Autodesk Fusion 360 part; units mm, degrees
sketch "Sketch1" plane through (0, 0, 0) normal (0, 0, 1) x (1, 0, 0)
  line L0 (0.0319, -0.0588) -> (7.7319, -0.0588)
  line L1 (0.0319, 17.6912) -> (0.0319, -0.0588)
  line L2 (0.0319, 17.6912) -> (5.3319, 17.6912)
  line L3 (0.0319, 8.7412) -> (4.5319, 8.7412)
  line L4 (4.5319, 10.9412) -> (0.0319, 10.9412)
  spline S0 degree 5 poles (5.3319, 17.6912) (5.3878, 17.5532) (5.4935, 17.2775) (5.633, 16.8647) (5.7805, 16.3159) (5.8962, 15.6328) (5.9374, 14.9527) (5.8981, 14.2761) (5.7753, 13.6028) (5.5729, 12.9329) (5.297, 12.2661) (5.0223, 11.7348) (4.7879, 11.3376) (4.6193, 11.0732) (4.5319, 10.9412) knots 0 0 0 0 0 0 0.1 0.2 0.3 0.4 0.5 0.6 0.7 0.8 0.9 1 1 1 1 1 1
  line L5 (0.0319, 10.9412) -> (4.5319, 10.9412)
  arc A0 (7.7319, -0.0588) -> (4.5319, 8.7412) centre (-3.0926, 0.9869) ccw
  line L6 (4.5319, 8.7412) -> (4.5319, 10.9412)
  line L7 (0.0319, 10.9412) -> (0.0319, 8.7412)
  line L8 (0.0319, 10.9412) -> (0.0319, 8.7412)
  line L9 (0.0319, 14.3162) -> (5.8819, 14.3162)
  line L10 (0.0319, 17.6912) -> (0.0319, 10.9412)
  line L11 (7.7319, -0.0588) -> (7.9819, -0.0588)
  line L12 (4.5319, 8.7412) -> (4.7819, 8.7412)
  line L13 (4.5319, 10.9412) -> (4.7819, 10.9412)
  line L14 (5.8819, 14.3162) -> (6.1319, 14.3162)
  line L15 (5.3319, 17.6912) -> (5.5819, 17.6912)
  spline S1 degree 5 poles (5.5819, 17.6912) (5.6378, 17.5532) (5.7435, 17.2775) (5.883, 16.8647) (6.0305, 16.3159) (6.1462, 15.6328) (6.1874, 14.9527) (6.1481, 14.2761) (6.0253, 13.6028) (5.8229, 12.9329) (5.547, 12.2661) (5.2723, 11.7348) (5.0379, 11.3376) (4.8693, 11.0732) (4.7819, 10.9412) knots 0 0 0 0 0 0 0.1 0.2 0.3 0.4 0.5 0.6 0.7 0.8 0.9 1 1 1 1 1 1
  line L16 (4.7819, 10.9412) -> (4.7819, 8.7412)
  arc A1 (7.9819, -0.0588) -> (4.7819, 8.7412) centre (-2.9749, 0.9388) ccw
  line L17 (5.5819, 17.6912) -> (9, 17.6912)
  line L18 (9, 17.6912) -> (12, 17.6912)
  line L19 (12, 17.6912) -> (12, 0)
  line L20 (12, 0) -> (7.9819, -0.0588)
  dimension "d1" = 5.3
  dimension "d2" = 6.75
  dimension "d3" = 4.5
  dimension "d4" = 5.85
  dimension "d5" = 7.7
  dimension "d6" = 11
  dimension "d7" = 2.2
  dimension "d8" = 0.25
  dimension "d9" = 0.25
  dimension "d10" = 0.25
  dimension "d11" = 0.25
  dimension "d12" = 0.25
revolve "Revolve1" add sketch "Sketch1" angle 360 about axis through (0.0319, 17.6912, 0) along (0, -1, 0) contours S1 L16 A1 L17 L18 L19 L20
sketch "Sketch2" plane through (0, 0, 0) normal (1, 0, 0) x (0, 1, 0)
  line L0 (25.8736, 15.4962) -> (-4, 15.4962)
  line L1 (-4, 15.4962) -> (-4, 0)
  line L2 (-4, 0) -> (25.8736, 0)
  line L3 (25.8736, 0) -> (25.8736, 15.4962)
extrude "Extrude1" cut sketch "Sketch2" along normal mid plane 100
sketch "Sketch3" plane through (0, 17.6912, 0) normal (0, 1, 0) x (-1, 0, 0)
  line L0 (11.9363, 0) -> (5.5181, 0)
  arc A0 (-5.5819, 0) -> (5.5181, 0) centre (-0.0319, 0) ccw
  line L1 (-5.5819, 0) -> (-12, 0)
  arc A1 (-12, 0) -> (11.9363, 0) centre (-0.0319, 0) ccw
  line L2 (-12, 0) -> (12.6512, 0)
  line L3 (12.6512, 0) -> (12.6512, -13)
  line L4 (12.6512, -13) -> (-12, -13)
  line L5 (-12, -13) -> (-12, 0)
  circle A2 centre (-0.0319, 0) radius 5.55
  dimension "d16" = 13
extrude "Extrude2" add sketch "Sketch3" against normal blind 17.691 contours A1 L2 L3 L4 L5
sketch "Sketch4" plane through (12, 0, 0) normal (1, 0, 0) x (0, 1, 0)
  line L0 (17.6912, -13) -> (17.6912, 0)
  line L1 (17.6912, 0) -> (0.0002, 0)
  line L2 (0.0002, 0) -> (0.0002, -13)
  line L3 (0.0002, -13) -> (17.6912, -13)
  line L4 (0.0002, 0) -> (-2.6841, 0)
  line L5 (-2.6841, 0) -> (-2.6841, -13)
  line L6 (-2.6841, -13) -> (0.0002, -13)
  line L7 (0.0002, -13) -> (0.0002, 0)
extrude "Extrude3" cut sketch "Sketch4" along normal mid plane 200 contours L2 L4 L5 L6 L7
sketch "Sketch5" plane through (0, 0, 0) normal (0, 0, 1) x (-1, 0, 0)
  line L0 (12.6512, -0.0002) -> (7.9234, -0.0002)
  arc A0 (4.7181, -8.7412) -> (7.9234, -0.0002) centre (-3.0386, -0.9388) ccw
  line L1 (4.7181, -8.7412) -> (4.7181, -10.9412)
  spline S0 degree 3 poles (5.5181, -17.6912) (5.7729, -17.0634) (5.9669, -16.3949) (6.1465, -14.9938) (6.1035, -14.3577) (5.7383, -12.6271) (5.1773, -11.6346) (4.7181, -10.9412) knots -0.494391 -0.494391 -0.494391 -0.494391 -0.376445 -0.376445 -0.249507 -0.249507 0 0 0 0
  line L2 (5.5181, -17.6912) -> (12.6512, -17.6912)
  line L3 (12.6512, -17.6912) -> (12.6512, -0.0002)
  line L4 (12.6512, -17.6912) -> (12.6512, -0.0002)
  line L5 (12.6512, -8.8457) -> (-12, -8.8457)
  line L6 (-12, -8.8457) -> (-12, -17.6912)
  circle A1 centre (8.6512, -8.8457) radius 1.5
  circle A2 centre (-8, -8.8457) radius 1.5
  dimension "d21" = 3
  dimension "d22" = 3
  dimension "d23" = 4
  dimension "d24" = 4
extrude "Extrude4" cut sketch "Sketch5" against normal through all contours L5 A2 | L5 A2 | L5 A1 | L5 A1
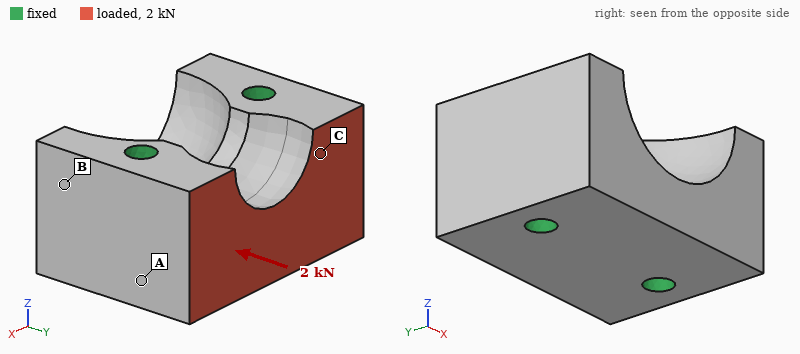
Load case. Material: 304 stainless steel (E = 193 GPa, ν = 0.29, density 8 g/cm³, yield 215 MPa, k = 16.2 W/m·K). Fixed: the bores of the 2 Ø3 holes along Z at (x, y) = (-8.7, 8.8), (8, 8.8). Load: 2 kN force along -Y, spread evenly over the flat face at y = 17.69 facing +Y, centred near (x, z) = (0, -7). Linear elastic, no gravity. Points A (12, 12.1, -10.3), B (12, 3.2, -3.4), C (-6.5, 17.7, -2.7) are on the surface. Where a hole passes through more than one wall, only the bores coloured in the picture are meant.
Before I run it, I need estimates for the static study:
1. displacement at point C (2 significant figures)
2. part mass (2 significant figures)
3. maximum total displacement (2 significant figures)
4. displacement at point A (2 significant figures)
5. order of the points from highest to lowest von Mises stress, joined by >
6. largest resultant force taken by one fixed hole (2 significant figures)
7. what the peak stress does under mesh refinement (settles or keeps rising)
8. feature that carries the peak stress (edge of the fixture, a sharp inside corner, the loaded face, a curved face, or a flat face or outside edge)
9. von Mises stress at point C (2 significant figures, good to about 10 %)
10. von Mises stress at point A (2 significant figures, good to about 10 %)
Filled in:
0.39 µm
35 g
0.56 µm
0.19 µm
C > A > B
1.0 kN
keeps rising
edge of the fixture
9.0 MPa
4.9 MPa
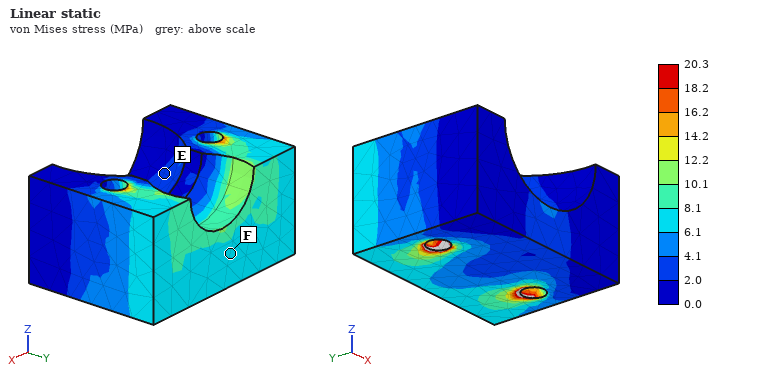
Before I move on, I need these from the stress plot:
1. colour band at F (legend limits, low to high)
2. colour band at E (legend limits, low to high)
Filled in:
6.1 to 8.1 MPa
2.0 to 4.1 MPa
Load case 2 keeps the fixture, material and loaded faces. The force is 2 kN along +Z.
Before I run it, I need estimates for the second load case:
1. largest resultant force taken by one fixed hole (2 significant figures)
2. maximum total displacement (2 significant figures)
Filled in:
1.0 kN
2.6 µm
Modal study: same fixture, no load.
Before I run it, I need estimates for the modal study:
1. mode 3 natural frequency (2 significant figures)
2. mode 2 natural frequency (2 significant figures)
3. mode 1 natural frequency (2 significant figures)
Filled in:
64 kHz
64 kHz
57 kHz
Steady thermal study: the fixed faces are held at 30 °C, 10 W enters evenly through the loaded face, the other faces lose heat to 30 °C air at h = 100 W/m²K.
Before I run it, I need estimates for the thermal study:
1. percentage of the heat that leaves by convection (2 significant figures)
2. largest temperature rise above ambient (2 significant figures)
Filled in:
8.4 %
22 K
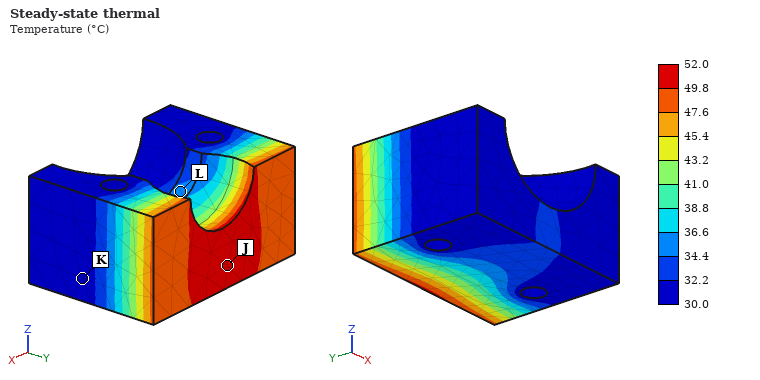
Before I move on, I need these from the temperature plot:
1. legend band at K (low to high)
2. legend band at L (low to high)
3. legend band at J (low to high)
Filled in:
30.0 to 32.2 °C
34.4 to 36.6 °C
49.8 to 52.0 °C
